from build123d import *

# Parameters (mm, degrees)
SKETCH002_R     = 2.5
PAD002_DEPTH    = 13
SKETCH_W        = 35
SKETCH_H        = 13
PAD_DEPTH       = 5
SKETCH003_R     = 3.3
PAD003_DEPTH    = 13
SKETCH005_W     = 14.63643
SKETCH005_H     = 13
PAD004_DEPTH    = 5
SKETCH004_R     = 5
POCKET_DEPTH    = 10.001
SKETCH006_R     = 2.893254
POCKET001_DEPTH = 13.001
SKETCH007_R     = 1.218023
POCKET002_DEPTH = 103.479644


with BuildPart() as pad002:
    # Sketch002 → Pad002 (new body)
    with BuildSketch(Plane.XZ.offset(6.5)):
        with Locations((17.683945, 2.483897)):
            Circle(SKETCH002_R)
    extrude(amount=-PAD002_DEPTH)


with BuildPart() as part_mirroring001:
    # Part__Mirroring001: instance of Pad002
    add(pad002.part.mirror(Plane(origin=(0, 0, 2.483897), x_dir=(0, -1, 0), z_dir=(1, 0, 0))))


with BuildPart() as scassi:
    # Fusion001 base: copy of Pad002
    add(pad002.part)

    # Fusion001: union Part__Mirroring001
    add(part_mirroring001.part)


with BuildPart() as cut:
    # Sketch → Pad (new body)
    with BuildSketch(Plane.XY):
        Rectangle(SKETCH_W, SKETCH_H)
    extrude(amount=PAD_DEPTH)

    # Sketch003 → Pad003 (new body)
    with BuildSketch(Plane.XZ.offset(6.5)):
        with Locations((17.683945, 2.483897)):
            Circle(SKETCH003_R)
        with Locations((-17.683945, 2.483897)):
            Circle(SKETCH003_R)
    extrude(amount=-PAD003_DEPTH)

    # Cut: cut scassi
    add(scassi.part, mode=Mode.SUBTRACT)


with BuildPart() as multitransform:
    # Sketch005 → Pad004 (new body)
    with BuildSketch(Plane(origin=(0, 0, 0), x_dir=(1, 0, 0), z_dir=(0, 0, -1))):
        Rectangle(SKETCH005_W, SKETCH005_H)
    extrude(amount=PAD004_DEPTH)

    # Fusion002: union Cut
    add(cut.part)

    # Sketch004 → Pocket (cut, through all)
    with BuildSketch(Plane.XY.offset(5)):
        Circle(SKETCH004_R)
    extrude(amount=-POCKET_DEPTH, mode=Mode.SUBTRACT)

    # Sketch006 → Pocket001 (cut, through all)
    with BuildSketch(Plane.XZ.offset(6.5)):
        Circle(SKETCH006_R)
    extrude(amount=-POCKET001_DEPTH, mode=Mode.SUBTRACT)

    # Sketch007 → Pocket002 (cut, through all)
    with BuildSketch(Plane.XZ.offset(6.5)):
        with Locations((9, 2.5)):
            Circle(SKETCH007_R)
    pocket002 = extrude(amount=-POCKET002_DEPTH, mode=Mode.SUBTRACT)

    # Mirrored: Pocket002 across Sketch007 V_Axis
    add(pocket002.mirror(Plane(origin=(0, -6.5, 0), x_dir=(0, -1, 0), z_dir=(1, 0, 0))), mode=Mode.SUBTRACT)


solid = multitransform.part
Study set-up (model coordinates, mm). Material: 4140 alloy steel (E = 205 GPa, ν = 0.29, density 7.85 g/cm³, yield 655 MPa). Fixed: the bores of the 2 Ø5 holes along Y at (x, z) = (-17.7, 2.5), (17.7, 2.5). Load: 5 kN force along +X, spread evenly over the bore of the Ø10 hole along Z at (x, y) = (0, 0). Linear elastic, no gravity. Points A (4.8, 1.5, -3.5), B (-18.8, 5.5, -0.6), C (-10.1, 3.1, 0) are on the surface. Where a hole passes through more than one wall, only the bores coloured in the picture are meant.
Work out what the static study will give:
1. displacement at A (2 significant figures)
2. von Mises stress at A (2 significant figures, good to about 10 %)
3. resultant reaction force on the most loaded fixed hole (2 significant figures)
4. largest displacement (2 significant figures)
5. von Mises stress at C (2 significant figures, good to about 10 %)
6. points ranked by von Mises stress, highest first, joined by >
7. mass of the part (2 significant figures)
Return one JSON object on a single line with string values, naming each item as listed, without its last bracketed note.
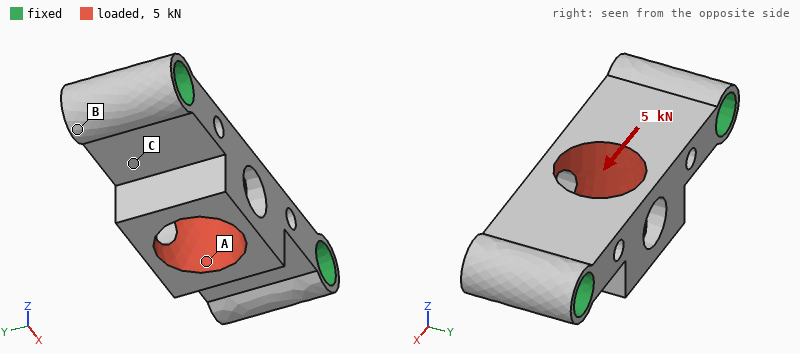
{"displacement at A": "7.7 µm", "von Mises stress at A": "33 MPa", "resultant reaction force on the most loaded fixed hole": "2.5 kN", "largest displacement": "9.5 µm", "von Mises stress at C": "74 MPa", "points ranked by von Mises stress, highest first, joined by >": "C > A > B", "mass of the part": "18 g"}
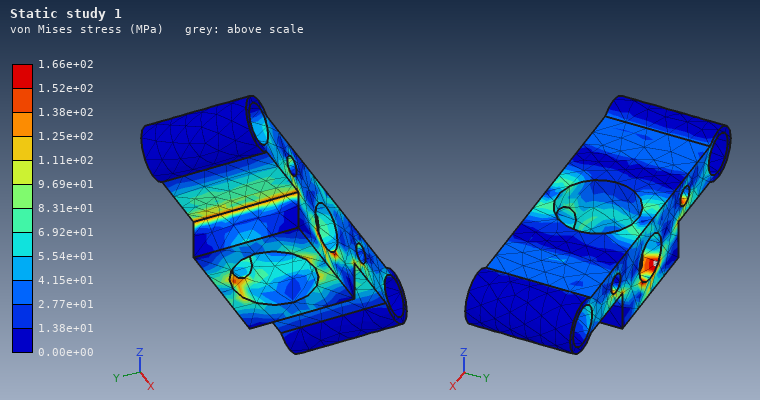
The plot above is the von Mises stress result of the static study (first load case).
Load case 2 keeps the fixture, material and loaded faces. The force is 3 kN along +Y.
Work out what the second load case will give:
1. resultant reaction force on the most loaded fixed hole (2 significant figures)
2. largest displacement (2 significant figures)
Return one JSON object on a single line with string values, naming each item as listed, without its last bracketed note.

{"resultant reaction force on the most loaded fixed hole": "1.5 kN", "largest displacement": "18 µm"}
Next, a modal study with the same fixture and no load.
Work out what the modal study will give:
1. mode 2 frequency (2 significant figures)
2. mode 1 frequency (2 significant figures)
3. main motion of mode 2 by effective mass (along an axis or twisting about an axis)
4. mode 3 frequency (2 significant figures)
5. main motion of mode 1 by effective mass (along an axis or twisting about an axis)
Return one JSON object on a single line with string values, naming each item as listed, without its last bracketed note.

{"mode 2 frequency": "24 kHz", "mode 1 frequency": "23 kHz", "main motion of mode 2 by effective mass": "along Y", "mode 3 frequency": "37 kHz", "main motion of mode 1 by effective mass": "along Z"}
